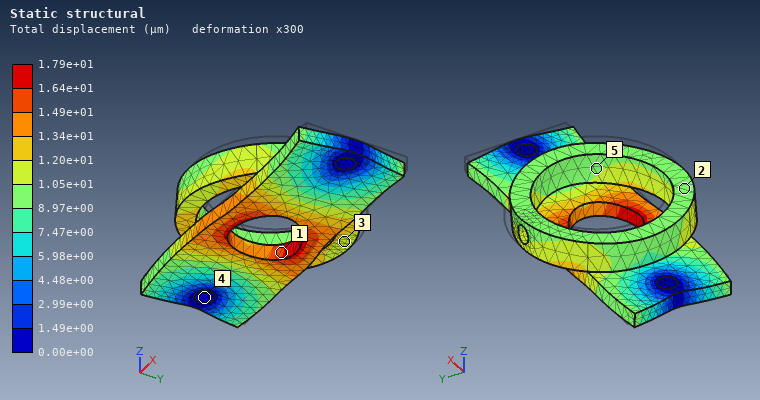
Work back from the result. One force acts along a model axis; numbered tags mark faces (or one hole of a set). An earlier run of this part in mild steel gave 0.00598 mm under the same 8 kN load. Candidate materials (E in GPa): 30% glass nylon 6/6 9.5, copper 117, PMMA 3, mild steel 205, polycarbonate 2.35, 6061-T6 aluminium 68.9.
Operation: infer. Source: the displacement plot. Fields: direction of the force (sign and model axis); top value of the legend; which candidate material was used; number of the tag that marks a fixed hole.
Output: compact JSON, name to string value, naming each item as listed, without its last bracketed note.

{"direction of the force": "-X", "top value of the legend": "1.79e+01 µm", "which candidate material was used": "6061-T6 aluminium", "number of the tag that marks a fixed hole": "4"}
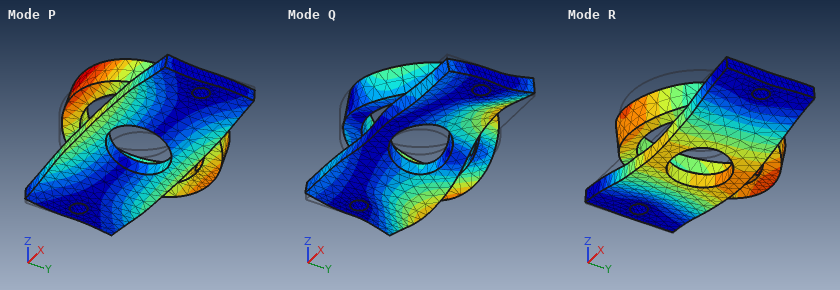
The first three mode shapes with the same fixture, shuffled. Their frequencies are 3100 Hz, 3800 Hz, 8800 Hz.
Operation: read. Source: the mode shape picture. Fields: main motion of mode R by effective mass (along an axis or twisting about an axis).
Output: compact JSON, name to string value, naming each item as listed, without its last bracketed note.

{"main motion of mode R by effective mass": "along Z"}
